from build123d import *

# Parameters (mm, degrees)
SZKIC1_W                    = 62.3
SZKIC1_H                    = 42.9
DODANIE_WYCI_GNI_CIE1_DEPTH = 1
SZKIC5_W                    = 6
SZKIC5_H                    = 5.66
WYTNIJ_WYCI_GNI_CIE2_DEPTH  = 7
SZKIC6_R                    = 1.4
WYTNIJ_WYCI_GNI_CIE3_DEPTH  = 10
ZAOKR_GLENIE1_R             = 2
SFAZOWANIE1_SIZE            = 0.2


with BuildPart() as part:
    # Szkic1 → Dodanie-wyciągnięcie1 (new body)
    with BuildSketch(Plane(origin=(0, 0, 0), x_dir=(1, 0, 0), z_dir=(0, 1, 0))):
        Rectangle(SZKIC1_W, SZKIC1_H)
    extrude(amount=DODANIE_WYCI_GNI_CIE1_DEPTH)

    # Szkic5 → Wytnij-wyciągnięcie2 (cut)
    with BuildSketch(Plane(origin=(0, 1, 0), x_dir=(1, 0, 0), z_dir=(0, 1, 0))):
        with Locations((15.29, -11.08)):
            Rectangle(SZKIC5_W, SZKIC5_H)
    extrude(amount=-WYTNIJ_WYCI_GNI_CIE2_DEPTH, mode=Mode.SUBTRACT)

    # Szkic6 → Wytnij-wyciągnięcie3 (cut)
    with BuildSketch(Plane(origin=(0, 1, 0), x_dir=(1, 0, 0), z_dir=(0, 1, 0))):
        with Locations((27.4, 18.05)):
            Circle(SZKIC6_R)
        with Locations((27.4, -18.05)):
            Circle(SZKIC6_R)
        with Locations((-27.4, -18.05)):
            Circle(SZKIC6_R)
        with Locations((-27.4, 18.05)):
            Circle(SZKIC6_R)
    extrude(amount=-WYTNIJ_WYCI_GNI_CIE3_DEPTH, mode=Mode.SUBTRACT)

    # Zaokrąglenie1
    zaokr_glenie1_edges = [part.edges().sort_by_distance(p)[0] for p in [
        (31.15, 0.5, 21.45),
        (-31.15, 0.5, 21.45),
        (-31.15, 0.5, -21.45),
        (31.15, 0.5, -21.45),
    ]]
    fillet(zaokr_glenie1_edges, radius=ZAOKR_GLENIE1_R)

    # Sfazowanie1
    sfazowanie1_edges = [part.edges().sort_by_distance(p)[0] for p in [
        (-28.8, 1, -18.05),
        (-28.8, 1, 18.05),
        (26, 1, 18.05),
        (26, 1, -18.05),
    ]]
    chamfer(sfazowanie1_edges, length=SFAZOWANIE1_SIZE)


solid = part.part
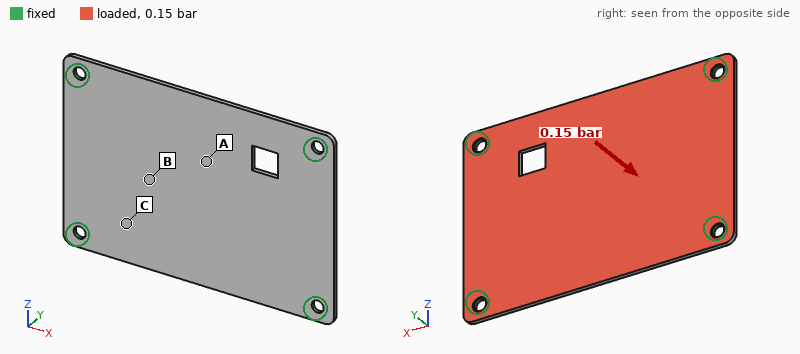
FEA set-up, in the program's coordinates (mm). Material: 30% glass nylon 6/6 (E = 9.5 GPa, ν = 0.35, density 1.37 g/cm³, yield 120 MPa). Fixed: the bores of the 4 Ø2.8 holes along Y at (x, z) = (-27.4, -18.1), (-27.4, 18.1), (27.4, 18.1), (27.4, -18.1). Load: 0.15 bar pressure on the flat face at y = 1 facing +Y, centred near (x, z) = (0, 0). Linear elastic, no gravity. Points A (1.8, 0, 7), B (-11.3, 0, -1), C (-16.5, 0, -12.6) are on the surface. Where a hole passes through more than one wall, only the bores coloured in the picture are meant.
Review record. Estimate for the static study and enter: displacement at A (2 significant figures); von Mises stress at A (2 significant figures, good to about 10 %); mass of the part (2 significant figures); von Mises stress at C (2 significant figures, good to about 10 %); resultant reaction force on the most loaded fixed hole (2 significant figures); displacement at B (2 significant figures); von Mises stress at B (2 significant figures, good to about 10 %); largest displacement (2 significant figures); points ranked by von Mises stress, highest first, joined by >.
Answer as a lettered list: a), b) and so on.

a) 0.59 mm
b) 11 MPa
c) 3.6 g
d) 3.4 MPa
e) 10.0 N
f) 0.48 mm
g) 7.7 MPa
h) 0.61 mm
i) A > B > C
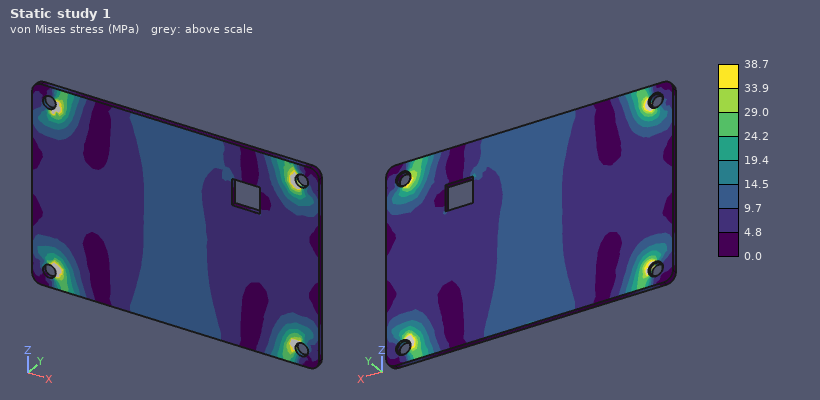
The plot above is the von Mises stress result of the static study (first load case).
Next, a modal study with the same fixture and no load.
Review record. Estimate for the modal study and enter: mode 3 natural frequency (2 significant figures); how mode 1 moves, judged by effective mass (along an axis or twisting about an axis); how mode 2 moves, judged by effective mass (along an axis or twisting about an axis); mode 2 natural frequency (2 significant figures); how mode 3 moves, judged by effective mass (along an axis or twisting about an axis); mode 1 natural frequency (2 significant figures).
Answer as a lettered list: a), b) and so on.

a) 1900 Hz
b) along Y
c) twisting about X
d) 1200 Hz
e) twisting about Z
f) 780 Hz
